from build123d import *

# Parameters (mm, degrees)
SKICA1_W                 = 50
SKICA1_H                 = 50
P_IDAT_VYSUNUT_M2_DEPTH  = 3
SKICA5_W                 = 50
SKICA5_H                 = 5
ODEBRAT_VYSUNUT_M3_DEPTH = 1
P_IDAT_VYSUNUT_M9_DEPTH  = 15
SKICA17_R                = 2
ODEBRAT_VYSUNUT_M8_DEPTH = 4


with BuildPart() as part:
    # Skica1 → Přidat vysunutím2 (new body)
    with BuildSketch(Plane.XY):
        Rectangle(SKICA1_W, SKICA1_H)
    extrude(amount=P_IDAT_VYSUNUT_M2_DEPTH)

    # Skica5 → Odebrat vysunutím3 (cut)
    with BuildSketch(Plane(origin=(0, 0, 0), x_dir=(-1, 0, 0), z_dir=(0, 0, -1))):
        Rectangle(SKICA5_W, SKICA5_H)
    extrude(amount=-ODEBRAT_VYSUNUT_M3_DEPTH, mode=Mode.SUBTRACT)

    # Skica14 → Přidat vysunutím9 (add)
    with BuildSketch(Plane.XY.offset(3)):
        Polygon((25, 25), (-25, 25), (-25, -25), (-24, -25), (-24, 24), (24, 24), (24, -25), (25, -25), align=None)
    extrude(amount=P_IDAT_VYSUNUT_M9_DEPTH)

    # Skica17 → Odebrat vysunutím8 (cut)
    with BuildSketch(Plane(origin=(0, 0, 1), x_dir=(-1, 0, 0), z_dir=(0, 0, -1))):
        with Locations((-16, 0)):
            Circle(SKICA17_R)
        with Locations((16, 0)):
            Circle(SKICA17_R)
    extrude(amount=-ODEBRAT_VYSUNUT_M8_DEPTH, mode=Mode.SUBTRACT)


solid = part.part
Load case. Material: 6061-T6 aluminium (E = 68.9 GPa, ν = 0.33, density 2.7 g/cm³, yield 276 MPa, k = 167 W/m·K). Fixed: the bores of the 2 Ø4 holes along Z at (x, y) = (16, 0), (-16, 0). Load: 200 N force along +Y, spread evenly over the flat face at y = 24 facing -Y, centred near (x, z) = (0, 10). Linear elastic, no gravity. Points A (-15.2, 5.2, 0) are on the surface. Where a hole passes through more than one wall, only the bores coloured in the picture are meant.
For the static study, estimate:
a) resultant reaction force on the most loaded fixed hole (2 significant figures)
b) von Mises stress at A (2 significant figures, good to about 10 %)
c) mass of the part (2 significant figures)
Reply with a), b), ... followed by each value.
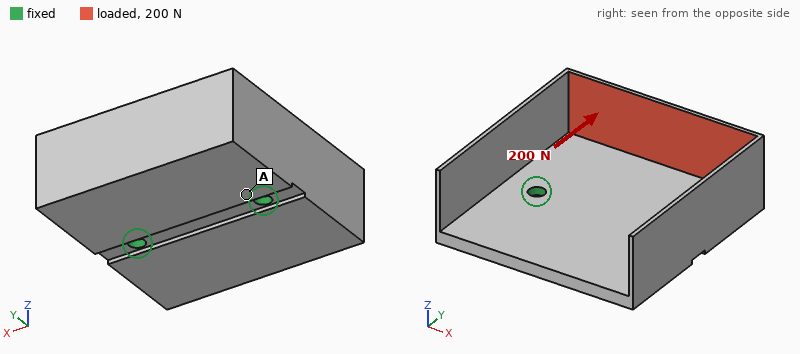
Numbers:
a) 100 N
b) 14 MPa
c) 25 g
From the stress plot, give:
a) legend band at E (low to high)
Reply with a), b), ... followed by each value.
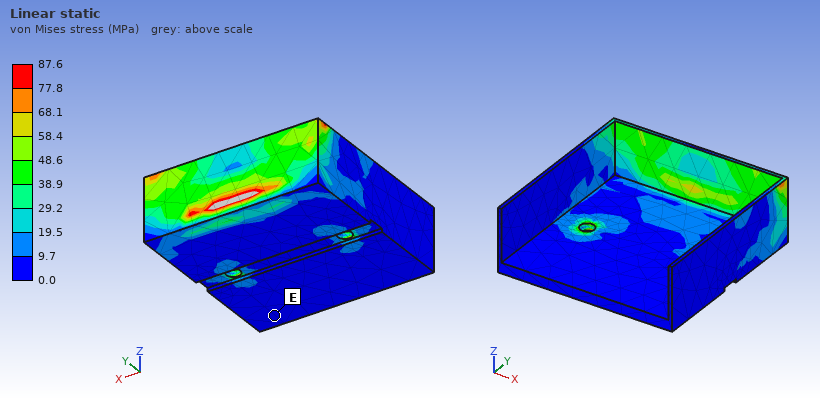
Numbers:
a) 0.0 to 9.7 MPa
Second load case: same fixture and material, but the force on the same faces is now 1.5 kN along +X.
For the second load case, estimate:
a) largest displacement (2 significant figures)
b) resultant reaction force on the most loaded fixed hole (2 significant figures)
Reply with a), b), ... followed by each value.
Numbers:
a) 0.41 mm
b) 1.3 kN
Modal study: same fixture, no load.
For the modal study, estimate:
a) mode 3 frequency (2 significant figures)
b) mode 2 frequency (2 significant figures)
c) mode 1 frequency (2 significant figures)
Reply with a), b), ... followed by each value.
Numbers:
a) 3700 Hz
b) 3200 Hz
c) 2200 Hz
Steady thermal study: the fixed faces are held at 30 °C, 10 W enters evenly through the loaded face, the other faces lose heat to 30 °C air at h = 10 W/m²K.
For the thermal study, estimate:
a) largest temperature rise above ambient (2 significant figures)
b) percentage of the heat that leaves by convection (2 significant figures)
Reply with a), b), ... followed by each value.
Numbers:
a) 18 K
b) 4.8 %
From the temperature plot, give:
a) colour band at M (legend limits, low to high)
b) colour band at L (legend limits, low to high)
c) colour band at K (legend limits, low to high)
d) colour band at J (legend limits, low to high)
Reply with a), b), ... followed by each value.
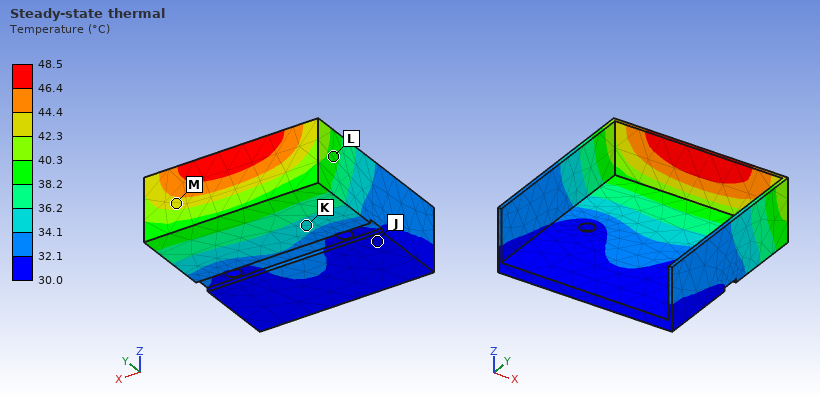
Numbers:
a) 42.3 to 44.4 °C
b) 38.2 to 40.3 °C
c) 34.1 to 36.2 °C
d) 30.0 to 32.1 °C
